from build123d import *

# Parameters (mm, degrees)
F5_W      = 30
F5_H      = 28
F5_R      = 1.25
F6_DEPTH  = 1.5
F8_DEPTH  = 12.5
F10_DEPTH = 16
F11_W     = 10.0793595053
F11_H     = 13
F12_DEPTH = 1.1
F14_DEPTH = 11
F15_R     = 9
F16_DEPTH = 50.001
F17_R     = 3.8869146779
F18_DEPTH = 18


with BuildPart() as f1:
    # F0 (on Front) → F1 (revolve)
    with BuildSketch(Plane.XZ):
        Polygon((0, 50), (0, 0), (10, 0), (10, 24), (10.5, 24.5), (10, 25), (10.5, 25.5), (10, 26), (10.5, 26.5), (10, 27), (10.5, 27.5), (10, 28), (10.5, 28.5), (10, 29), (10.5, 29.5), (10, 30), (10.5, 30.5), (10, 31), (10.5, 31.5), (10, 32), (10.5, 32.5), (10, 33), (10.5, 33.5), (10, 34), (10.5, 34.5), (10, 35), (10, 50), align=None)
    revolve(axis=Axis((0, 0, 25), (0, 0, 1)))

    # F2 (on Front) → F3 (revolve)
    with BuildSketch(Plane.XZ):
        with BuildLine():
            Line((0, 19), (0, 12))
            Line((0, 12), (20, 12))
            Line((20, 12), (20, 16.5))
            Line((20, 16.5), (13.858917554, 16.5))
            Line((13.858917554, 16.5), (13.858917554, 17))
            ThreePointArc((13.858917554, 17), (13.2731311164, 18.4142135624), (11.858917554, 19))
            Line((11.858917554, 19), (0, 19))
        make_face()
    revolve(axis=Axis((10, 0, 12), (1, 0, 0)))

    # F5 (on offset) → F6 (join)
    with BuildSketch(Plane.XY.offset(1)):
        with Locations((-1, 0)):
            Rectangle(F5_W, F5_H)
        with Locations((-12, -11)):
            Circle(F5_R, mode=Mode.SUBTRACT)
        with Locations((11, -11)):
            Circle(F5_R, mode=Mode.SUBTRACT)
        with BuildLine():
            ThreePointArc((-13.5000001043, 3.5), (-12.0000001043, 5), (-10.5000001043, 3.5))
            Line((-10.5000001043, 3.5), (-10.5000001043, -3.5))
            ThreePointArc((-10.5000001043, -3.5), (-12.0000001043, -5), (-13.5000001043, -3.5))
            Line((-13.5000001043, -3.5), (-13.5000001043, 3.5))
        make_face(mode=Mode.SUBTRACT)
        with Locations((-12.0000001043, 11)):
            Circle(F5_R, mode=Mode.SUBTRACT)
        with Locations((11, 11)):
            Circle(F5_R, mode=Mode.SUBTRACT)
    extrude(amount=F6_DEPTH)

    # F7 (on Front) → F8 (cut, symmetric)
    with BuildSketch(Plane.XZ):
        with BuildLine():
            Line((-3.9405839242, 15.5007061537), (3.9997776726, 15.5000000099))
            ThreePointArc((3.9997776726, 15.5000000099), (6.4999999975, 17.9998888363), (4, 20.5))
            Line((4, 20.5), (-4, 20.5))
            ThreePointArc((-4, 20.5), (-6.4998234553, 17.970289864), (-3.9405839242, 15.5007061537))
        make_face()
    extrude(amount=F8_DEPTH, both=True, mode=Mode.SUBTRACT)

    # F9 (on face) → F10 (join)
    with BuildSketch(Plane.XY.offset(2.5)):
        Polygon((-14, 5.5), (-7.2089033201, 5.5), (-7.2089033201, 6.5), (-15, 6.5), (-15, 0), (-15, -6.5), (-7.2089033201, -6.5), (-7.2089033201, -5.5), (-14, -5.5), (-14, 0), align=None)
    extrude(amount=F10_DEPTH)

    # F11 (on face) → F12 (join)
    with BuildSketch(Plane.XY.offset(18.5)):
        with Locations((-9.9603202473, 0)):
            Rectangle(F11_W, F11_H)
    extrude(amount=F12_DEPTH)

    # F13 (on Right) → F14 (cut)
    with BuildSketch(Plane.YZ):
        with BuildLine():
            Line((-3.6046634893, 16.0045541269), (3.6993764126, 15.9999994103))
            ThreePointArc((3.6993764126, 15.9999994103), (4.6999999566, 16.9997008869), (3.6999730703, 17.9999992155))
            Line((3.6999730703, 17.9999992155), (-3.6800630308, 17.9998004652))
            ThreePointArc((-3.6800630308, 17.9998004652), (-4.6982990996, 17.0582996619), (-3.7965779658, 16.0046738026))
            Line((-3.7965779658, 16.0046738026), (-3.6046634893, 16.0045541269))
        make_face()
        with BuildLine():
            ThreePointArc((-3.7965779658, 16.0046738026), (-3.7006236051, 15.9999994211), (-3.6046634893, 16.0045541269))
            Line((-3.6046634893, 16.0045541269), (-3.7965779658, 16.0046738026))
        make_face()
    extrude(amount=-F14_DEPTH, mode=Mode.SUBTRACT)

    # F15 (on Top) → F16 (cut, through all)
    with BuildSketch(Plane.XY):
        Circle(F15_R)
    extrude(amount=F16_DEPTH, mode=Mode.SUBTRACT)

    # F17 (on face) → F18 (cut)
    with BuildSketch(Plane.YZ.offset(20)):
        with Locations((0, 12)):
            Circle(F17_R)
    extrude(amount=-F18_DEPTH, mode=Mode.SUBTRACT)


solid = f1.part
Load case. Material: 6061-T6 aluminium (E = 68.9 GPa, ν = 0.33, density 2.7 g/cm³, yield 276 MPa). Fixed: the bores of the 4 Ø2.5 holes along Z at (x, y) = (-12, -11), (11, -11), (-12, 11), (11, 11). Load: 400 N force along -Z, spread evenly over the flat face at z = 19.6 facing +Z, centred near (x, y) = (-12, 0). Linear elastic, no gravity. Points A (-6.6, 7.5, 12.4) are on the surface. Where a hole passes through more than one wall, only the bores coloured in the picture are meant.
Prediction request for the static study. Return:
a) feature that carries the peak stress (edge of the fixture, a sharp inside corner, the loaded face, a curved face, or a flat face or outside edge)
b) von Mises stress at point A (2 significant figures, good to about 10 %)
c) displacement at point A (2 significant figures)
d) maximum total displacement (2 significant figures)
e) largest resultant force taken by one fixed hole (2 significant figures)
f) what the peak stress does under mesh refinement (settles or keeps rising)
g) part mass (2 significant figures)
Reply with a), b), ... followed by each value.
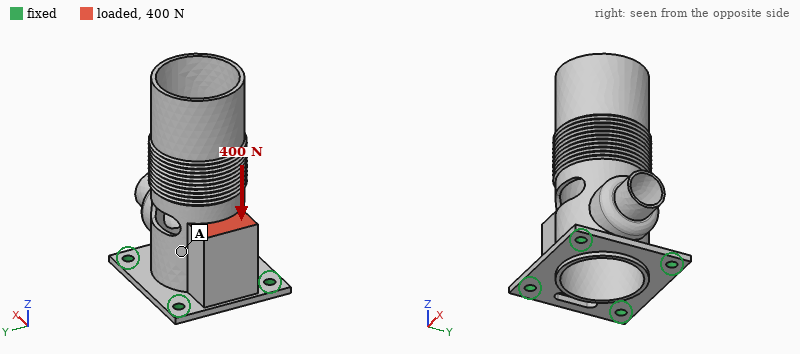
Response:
a) edge of the fixture
b) 9.4 MPa
c) 15 µm
d) 50 µm
e) 210 N
f) keeps rising
g) 13 g
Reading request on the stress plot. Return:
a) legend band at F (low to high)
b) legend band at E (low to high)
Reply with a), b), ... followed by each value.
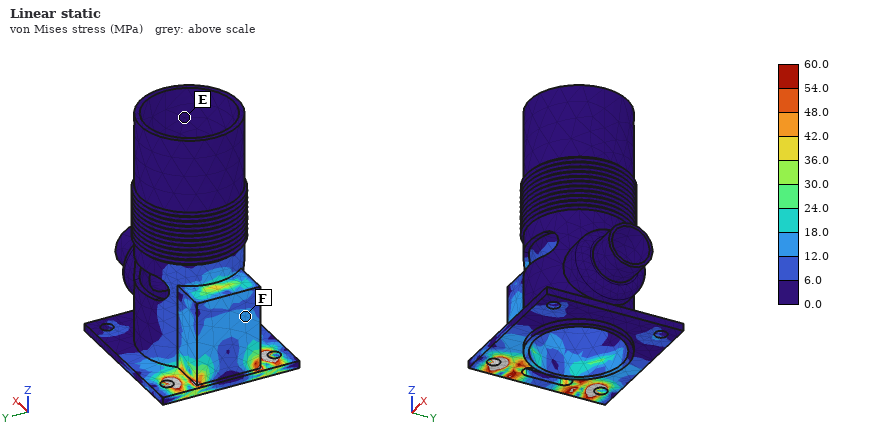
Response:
a) 12.0 to 18.0 MPa
b) 0.0 to 6.0 MPa
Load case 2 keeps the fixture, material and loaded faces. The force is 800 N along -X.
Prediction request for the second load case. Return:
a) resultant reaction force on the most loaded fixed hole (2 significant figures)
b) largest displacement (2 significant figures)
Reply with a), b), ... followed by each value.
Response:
a) 400 N
b) 0.21 mm
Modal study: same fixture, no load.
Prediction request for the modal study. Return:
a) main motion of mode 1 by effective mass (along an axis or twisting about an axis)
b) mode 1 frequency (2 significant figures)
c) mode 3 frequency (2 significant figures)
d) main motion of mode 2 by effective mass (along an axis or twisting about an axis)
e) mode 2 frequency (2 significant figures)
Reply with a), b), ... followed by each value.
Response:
a) along Y
b) 2800 Hz
c) 8000 Hz
d) along X
e) 3100 Hz
